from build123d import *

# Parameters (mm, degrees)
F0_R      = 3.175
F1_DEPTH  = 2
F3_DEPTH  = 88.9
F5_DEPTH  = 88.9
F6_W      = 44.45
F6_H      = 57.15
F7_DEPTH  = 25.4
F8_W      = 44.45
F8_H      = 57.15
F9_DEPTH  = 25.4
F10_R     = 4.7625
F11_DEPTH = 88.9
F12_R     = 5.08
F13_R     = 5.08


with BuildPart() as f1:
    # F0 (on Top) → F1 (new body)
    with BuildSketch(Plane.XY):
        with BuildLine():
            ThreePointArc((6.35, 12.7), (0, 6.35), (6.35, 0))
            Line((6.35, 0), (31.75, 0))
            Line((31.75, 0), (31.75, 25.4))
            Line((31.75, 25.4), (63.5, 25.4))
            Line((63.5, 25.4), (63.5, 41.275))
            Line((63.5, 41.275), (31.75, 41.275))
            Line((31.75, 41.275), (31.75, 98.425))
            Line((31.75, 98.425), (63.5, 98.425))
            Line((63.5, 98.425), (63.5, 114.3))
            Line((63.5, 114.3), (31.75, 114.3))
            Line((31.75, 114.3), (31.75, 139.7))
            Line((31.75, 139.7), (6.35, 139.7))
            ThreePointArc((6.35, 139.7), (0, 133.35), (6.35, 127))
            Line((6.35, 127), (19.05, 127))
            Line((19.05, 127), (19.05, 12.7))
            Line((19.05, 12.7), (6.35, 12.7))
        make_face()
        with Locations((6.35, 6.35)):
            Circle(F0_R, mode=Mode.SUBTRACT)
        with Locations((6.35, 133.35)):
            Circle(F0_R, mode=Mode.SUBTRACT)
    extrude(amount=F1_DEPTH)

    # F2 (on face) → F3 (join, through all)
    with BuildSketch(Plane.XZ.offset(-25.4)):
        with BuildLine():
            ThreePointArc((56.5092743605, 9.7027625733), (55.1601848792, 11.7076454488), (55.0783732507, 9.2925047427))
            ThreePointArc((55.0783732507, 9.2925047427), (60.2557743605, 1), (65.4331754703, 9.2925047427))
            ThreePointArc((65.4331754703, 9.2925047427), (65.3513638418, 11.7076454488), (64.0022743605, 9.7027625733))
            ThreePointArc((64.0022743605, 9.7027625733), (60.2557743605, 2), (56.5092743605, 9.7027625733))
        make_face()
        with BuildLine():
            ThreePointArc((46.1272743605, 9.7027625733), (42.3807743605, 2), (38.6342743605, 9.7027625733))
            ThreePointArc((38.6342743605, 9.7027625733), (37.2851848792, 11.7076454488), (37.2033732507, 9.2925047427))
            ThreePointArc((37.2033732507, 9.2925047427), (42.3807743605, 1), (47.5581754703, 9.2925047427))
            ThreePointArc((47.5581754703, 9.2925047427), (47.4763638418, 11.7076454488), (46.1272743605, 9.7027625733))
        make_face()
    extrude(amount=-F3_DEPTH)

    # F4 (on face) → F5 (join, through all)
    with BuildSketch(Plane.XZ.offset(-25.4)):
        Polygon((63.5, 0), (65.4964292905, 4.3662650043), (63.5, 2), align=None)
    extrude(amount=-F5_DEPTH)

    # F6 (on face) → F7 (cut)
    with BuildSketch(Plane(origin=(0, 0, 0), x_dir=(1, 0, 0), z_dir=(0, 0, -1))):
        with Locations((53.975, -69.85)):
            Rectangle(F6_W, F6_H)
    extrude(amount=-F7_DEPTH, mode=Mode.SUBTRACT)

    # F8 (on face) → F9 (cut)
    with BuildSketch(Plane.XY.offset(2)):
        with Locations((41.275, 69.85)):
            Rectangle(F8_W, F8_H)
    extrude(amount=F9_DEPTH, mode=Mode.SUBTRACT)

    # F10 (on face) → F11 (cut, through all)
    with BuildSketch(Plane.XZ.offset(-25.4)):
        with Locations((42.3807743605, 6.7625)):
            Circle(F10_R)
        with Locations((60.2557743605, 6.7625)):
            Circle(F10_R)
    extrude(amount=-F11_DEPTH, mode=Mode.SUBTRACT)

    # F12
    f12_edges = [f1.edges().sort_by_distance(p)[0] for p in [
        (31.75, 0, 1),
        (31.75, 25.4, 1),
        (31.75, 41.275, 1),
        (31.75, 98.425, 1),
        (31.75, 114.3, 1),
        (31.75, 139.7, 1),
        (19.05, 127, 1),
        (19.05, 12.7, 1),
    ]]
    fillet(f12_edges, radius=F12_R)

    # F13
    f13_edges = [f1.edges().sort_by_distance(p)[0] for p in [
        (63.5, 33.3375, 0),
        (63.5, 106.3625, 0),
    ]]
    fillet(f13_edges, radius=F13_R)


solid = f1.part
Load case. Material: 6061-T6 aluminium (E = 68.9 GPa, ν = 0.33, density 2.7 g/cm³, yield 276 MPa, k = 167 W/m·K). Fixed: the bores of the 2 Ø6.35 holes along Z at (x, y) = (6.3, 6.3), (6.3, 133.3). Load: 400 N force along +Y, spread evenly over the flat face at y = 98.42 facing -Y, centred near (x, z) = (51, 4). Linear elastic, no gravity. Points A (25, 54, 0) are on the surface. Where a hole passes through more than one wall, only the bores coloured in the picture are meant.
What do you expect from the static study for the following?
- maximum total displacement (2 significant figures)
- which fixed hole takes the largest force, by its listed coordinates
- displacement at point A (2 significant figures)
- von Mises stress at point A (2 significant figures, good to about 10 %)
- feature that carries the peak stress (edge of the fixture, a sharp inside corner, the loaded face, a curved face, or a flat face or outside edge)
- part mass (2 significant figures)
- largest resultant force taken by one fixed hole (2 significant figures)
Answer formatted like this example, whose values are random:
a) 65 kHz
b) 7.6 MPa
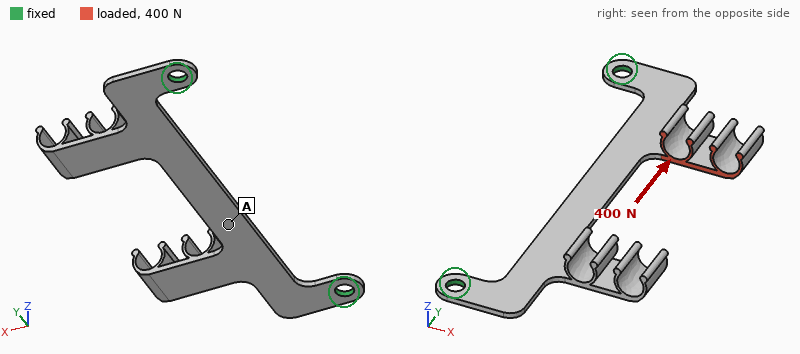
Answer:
a) 0.99 mm
b) (6.3, 6.3)
c) 0.50 mm
d) 14 MPa
e) a curved face
f) 22 g
g) 340 N
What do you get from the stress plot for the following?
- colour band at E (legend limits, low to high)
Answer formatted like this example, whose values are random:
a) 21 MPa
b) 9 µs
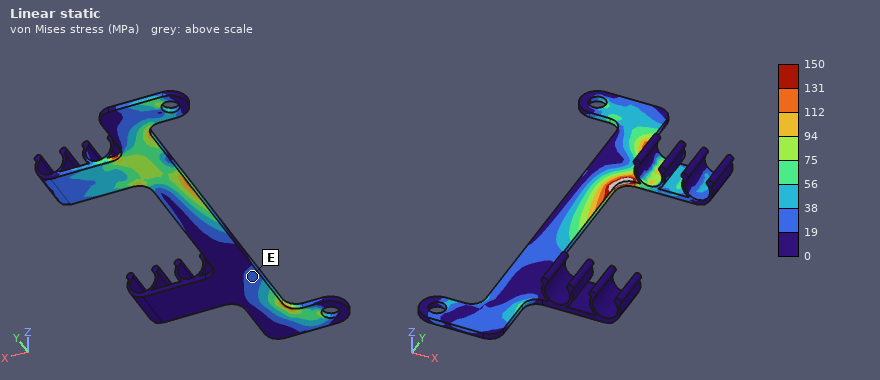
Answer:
a) 19 to 38 MPa
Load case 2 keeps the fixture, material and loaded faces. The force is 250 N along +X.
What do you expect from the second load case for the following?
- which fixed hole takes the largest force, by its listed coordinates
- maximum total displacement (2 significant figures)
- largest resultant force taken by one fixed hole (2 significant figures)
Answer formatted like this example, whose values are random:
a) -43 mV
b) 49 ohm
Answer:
a) (6.3, 133.3)
b) 1.8 mm
c) 250 N
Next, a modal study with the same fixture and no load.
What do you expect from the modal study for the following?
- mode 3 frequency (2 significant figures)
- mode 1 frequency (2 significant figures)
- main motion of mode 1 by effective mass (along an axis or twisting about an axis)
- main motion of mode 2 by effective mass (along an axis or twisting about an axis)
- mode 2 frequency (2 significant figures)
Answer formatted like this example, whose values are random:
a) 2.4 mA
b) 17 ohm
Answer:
a) 660 Hz
b) 270 Hz
c) along Z
d) twisting about X
e) 420 Hz
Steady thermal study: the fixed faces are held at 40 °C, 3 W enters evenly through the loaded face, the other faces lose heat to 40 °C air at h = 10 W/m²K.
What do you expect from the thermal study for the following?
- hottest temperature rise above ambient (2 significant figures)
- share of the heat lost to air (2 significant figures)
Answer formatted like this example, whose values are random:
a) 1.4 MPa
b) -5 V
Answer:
a) 24 K
b) 30 %
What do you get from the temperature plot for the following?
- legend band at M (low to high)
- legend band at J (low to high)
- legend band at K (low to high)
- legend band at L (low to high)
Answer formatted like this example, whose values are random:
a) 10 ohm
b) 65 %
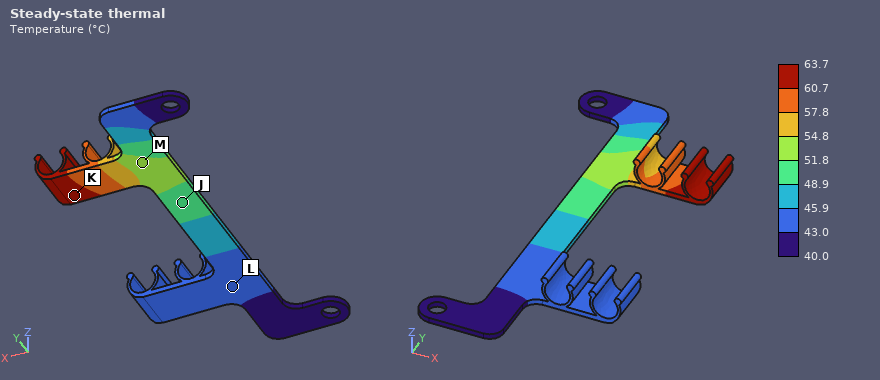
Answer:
a) 51.8 to 54.8 °C
b) 48.9 to 51.8 °C
c) 60.7 to 63.7 °C
d) 43.0 to 45.9 °C
